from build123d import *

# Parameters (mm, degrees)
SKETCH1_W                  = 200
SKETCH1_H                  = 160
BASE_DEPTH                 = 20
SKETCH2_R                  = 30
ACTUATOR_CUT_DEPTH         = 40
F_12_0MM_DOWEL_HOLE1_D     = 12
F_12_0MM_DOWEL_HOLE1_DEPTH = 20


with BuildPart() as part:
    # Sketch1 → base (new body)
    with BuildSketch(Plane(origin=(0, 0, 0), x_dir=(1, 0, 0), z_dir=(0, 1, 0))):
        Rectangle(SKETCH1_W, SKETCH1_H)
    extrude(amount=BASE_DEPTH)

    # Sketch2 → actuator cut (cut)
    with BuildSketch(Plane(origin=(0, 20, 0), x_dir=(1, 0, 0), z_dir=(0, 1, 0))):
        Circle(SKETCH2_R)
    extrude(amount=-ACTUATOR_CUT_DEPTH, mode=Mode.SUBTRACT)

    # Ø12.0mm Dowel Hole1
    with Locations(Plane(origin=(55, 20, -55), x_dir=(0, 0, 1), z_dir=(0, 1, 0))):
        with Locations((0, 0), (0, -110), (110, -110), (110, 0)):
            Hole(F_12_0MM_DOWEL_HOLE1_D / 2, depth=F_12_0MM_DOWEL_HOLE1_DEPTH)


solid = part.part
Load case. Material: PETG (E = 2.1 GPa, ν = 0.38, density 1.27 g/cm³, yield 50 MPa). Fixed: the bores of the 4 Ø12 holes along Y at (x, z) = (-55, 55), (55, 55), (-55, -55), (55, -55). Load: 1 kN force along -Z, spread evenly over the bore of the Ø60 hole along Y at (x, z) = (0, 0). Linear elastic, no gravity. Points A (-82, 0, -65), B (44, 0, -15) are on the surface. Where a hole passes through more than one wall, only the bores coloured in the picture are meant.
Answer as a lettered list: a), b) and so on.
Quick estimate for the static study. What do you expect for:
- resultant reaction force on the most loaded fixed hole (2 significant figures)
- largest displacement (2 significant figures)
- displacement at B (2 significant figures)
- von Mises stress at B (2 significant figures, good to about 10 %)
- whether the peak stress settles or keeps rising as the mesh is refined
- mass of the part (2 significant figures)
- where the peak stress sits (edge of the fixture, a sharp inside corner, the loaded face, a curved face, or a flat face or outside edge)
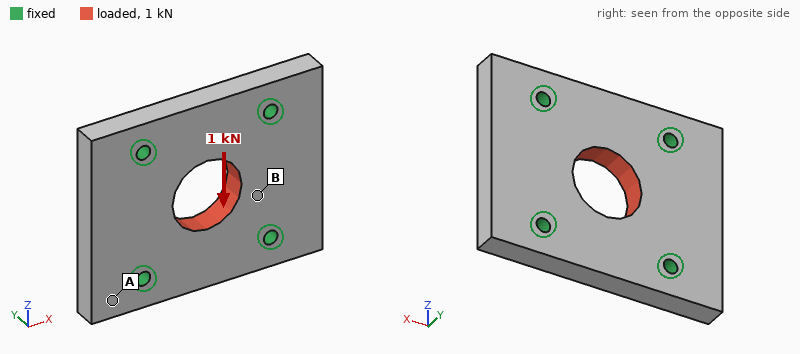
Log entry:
a) 270 N
b) 13 µm
c) 5.2 µm
d) 0.28 MPa
e) keeps rising
f) 730 g
g) edge of the fixture
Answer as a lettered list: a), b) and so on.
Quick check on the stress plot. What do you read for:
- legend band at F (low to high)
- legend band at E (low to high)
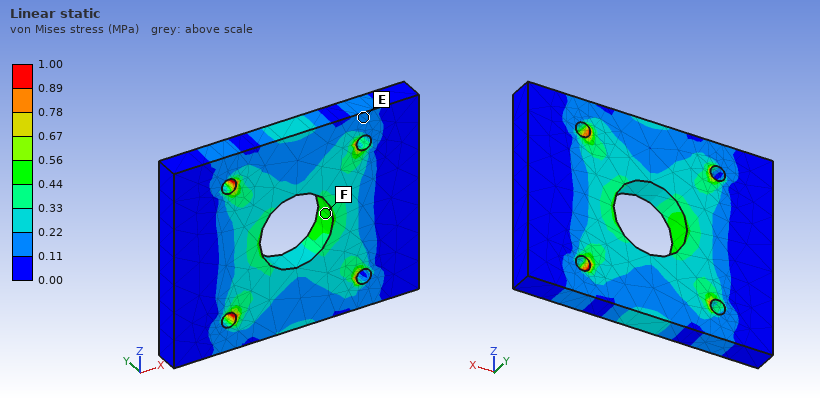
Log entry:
a) 0.44 to 0.56 MPa
b) 0.11 to 0.22 MPa
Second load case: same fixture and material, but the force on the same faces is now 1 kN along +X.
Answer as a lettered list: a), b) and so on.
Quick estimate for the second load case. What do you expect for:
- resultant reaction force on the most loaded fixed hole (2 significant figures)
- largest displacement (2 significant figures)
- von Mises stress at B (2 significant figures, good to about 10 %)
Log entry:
a) 260 N
b) 11 µm
c) 0.21 MPa
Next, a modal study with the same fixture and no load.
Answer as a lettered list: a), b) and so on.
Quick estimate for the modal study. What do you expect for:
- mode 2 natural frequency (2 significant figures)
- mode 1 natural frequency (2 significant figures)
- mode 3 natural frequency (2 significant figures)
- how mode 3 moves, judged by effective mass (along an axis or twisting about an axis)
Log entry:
a) 1300 Hz
b) 1300 Hz
c) 1500 Hz
d) along Y
